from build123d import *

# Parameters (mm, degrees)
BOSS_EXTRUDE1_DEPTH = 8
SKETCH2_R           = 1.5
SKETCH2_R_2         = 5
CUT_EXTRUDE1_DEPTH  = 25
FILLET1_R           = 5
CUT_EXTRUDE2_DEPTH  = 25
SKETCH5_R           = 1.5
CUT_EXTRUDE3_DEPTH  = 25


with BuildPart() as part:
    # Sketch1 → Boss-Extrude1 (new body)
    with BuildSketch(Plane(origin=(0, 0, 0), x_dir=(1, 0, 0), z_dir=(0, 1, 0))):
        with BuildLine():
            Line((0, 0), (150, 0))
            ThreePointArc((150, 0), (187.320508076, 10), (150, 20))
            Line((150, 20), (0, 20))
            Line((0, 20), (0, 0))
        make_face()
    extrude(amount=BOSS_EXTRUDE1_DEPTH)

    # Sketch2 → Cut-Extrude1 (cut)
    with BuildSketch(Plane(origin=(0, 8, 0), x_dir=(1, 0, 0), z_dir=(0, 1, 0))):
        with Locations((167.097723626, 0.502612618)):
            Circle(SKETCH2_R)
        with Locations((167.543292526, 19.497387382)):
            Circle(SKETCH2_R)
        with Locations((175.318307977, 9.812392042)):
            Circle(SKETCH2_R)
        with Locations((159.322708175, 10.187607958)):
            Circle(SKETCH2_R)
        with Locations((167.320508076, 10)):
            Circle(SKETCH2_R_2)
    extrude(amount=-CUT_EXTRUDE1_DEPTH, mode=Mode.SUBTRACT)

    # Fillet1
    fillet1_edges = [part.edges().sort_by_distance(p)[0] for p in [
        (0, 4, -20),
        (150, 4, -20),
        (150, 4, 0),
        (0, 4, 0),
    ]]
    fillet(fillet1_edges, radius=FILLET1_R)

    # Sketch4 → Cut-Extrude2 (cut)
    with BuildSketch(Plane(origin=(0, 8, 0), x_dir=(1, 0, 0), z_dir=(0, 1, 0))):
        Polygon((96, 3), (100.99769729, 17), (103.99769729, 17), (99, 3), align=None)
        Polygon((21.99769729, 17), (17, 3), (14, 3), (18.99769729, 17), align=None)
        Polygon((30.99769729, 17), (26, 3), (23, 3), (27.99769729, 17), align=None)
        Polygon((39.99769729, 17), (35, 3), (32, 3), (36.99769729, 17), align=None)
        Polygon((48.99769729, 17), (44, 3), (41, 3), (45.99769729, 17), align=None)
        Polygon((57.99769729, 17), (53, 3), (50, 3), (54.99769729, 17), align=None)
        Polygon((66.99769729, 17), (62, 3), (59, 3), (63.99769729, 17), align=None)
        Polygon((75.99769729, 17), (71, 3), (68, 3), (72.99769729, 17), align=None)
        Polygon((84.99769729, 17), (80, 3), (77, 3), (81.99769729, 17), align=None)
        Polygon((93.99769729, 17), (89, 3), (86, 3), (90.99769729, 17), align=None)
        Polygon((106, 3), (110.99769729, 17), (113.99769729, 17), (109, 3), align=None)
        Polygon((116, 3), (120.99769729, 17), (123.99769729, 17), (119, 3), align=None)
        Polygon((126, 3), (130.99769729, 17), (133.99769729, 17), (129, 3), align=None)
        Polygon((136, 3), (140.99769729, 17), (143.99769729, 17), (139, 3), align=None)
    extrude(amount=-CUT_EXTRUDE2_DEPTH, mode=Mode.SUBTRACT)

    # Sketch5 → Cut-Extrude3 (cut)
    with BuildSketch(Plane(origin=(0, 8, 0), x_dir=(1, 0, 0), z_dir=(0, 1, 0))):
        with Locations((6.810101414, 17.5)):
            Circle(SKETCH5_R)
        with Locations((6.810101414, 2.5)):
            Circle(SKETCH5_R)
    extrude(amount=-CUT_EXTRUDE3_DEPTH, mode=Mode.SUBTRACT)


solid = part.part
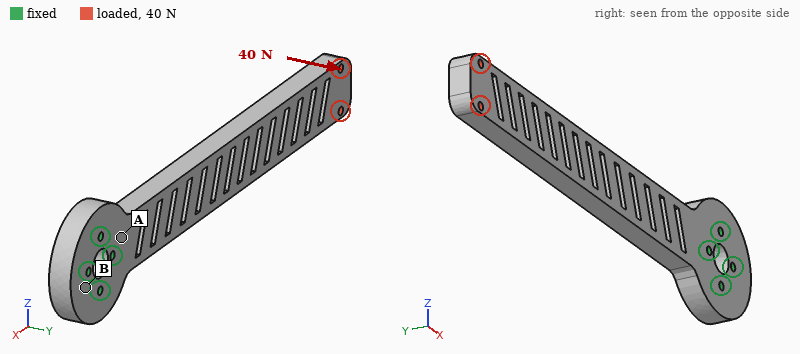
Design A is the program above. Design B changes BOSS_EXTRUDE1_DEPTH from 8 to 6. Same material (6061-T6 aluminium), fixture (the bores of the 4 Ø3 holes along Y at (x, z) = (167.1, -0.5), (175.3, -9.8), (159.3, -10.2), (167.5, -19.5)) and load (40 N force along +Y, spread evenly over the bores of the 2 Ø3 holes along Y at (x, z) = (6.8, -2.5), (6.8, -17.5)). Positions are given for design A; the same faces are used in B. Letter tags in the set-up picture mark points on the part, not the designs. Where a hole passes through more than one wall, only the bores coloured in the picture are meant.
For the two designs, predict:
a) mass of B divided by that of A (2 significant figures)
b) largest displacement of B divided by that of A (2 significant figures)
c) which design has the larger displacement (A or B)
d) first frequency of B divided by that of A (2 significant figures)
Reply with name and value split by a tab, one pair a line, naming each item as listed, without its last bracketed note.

mass of B divided by that of A	0.75
largest displacement of B divided by that of A	2.3
which design has the larger displacement	B
first frequency of B divided by that of A	0.76
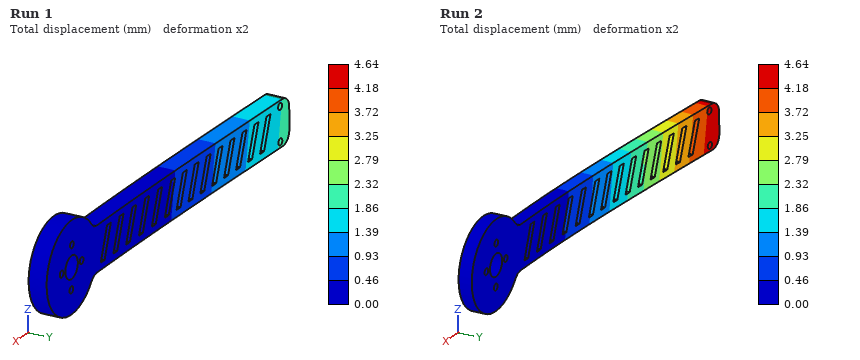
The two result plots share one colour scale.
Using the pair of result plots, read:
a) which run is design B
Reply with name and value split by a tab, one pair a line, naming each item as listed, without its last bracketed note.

which run is design B	Run 2
